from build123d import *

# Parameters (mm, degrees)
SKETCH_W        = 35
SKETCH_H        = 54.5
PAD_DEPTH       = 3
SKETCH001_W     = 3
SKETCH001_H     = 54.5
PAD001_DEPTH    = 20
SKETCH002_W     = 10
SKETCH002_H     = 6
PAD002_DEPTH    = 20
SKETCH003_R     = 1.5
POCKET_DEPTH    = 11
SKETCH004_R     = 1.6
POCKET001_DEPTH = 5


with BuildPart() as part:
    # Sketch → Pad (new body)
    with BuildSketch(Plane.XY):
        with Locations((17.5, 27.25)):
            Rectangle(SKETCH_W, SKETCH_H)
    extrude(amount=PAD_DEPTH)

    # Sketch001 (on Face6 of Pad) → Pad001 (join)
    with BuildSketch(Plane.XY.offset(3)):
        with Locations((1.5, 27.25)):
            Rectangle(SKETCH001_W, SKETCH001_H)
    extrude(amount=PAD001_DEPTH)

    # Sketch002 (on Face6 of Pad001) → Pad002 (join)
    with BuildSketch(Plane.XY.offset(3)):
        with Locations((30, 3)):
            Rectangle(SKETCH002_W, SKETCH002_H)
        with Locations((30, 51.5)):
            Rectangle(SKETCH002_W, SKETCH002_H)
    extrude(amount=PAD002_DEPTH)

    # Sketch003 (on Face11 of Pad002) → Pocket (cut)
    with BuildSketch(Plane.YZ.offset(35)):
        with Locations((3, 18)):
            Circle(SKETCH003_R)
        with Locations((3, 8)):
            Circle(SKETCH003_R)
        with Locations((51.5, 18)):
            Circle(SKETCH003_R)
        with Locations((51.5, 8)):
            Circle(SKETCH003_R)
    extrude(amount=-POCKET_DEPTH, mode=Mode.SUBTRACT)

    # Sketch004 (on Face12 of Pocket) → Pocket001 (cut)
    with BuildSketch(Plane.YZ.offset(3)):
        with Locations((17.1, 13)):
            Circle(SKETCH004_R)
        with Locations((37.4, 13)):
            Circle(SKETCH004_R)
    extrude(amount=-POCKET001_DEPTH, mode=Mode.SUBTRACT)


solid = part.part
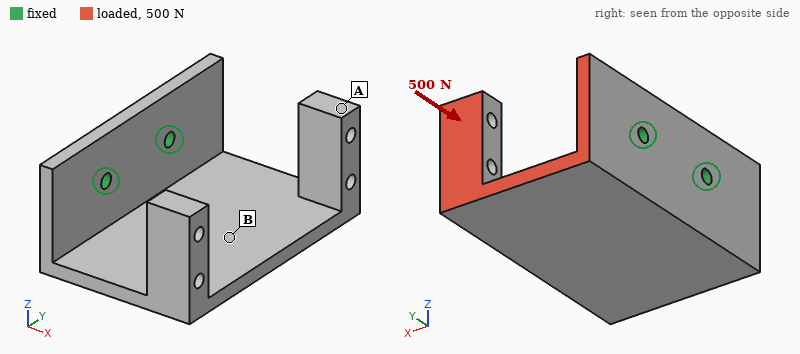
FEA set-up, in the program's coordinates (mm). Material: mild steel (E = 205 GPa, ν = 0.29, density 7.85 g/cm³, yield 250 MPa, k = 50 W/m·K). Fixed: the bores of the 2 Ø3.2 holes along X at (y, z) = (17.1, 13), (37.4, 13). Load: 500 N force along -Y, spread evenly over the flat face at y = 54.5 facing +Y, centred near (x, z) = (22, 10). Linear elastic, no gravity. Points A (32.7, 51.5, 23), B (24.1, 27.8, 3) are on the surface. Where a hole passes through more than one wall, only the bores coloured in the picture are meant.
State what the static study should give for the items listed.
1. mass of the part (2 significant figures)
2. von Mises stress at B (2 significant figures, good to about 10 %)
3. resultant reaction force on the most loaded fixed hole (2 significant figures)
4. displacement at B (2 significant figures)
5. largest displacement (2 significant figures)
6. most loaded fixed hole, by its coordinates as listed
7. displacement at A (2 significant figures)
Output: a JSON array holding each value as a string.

["87 g", "31 MPa", "500 N", "0.032 mm", "0.19 mm", "(37.4, 13)", "0.18 mm"]
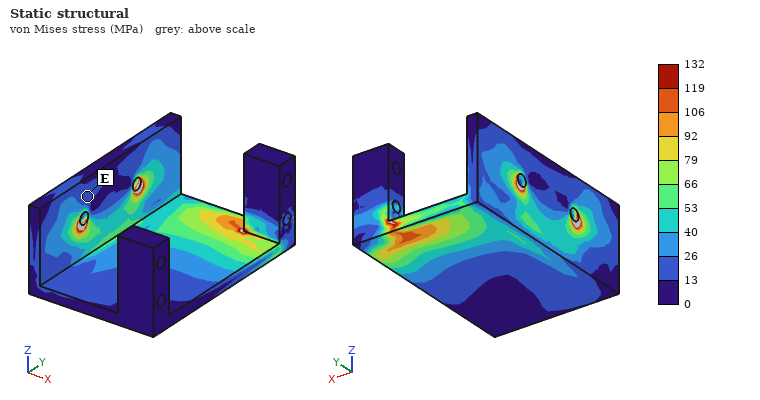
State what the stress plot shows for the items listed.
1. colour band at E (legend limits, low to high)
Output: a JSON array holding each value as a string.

["13 to 26 MPa"]
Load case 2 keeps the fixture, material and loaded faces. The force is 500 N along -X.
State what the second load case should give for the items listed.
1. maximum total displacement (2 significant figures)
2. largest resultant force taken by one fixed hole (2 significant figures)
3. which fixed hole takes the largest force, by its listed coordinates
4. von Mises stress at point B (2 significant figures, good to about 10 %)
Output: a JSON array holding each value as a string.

["0.19 mm", "760 N", "(37.4, 13)", "30 MPa"]
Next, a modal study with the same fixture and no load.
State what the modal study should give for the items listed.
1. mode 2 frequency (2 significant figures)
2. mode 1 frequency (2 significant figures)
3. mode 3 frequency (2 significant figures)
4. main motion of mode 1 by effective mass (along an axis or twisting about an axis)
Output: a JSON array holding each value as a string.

["1500 Hz", "970 Hz", "2300 Hz", "along Z"]
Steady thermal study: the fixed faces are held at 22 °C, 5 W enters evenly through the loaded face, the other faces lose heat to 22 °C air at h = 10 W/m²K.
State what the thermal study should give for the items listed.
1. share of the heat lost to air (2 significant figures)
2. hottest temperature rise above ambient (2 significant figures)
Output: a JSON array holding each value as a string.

["18 %", "43 K"]
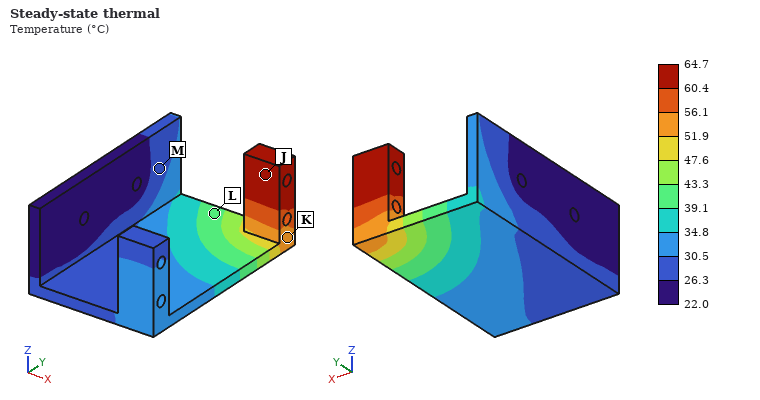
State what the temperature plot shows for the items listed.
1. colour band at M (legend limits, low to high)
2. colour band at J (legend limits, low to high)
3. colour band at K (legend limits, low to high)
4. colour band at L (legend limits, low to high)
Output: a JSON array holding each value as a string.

["26.3 to 30.5 °C", "60.4 to 64.7 °C", "51.9 to 56.1 °C", "39.1 to 43.3 °C"]
